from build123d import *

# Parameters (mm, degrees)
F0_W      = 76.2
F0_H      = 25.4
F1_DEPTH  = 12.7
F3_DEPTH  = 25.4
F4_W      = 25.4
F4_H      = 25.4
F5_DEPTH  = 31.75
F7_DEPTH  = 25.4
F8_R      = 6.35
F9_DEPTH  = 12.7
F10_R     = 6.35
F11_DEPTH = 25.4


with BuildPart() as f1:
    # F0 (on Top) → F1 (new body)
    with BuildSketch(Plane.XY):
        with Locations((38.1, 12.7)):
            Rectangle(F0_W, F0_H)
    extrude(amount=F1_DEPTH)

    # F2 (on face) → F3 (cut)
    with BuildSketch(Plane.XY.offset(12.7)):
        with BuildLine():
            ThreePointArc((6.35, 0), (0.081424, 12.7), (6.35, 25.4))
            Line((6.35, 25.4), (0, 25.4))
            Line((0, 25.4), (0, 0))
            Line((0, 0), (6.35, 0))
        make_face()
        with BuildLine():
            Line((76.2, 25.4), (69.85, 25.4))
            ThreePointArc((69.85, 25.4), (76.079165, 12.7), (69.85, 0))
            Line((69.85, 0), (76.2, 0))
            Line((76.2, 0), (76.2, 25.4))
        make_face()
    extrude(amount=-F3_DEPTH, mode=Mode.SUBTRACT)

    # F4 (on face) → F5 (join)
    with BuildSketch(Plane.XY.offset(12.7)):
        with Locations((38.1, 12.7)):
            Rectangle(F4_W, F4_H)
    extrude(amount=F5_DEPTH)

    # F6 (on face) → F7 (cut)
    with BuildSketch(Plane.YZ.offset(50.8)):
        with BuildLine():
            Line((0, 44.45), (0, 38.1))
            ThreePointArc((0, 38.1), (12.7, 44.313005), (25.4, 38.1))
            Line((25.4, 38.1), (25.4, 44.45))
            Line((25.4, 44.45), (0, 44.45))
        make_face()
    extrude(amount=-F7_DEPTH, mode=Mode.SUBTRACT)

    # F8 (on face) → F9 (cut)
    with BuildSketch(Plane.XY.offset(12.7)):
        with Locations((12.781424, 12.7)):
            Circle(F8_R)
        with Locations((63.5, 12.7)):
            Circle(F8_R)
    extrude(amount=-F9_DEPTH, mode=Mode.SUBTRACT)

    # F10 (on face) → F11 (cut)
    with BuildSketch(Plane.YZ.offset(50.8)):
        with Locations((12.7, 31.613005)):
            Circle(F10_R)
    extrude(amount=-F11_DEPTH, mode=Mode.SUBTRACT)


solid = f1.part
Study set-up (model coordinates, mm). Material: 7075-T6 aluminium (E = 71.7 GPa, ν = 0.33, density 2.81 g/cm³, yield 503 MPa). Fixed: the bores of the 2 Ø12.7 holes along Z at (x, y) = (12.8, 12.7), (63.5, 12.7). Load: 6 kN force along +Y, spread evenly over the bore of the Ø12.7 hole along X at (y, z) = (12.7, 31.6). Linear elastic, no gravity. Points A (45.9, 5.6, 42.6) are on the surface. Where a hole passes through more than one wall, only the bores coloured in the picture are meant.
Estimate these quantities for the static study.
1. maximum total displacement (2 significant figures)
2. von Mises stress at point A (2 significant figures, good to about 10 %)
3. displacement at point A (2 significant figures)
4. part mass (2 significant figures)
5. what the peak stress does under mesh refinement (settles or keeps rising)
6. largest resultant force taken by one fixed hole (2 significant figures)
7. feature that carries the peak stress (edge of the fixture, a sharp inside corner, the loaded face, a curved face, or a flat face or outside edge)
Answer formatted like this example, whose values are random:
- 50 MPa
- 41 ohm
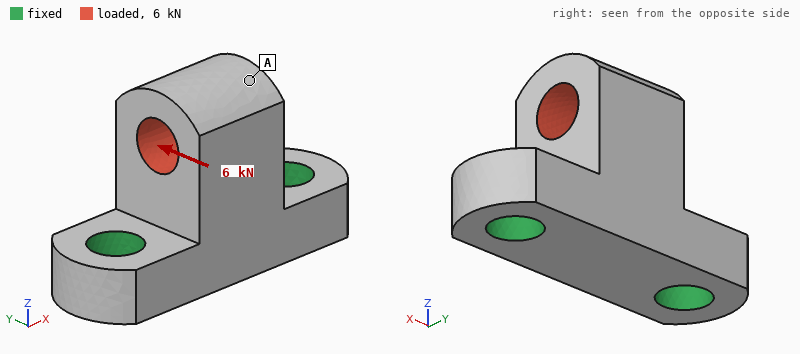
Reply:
- 0.13 mm
- 16 MPa
- 0.12 mm
- 100 g
- keeps rising
- 3.0 kN
- edge of the fixture
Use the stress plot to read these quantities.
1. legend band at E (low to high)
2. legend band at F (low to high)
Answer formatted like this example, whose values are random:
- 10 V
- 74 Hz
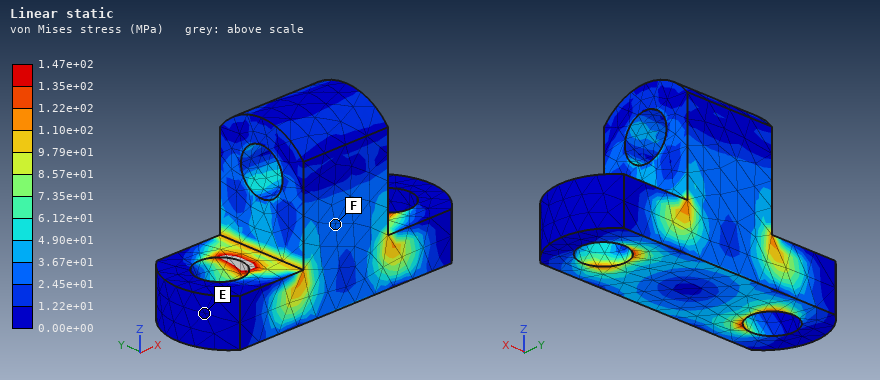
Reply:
- 0.00e+00 to 1.22e+01 MPa
- 2.45e+01 to 3.67e+01 MPa
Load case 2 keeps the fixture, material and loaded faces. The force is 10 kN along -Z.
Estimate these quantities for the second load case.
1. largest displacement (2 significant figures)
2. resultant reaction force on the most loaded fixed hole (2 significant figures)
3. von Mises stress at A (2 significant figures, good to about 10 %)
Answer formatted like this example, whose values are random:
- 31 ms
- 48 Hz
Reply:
- 22 µm
- 5.2 kN
- 11 MPa
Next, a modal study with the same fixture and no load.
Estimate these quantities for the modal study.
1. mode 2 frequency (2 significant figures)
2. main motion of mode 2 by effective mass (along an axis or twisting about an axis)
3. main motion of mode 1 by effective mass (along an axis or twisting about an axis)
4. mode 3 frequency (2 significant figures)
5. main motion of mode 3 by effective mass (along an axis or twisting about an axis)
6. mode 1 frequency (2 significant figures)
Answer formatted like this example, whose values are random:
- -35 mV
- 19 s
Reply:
- 12 kHz
- along X
- along Y
- 17 kHz
- along Z
- 6700 Hz
